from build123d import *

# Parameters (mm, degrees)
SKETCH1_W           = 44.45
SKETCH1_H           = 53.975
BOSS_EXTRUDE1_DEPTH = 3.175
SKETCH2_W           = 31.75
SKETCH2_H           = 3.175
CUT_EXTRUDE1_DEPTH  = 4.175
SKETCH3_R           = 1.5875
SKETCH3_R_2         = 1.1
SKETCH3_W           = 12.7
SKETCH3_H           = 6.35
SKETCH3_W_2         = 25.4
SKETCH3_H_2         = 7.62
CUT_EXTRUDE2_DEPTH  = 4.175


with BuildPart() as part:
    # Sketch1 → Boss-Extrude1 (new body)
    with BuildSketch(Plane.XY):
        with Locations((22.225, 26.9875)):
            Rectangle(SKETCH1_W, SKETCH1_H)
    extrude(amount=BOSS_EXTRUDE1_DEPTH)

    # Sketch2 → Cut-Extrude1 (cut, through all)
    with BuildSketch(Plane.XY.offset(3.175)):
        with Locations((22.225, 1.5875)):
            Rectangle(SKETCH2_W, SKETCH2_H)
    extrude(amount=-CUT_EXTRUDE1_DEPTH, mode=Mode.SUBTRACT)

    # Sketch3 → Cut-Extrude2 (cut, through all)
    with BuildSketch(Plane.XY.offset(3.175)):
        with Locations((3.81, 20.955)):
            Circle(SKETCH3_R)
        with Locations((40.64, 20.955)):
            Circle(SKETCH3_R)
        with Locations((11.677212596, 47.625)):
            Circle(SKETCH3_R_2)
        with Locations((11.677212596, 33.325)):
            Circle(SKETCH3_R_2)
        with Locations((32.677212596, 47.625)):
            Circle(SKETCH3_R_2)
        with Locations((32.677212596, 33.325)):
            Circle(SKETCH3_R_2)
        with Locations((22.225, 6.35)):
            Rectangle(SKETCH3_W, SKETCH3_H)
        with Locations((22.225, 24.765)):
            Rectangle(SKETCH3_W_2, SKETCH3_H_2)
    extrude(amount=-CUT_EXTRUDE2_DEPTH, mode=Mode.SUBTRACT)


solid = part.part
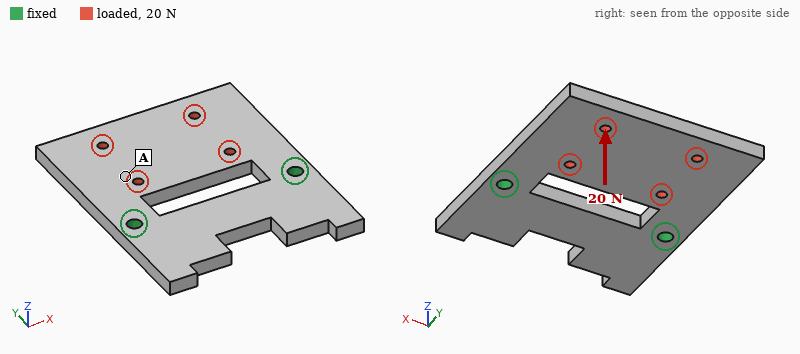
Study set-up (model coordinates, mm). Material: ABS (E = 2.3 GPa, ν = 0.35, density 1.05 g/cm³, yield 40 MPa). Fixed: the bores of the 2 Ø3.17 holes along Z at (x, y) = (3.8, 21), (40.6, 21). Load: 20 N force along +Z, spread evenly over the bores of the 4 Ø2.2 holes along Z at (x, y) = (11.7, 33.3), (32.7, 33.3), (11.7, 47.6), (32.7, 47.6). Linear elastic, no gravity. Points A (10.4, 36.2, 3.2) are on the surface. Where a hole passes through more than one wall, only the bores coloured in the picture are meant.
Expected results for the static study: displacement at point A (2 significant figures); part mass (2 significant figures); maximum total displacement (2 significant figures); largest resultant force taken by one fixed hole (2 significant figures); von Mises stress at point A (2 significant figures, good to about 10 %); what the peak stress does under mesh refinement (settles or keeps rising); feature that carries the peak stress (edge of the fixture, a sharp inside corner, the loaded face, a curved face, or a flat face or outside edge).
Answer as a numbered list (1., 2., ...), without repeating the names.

1. 0.28 mm
2. 6.6 g
3. 0.84 mm
4. 10 N
5. 1.9 MPa
6. keeps rising
7. edge of the fixture
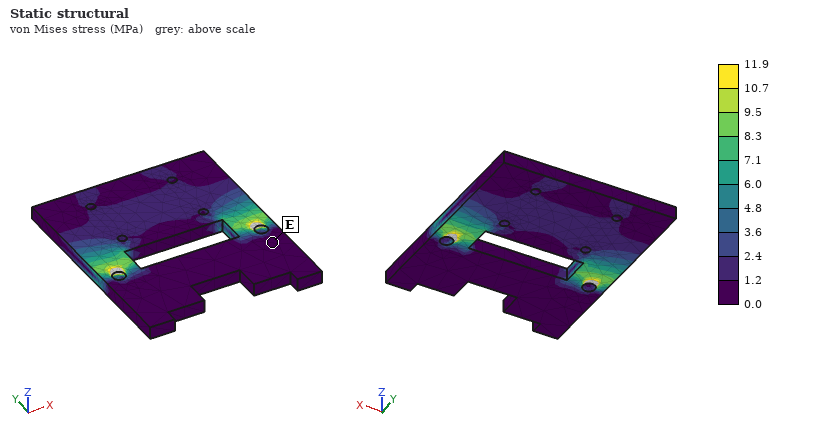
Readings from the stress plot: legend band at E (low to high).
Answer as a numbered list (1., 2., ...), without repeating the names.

1. 0.0 to 1.2 MPa
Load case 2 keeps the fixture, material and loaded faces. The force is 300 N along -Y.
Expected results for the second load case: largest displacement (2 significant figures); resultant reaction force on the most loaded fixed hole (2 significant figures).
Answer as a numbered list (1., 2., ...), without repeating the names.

1. 53 µm
2. 150 N
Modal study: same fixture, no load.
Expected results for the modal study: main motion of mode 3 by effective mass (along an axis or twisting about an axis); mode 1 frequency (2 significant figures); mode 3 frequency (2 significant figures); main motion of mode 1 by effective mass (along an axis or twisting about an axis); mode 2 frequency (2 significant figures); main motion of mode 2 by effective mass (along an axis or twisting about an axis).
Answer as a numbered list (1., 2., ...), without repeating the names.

1. along Z
2. 490 Hz
3. 1700 Hz
4. along Z
5. 1300 Hz
6. twisting about Y
